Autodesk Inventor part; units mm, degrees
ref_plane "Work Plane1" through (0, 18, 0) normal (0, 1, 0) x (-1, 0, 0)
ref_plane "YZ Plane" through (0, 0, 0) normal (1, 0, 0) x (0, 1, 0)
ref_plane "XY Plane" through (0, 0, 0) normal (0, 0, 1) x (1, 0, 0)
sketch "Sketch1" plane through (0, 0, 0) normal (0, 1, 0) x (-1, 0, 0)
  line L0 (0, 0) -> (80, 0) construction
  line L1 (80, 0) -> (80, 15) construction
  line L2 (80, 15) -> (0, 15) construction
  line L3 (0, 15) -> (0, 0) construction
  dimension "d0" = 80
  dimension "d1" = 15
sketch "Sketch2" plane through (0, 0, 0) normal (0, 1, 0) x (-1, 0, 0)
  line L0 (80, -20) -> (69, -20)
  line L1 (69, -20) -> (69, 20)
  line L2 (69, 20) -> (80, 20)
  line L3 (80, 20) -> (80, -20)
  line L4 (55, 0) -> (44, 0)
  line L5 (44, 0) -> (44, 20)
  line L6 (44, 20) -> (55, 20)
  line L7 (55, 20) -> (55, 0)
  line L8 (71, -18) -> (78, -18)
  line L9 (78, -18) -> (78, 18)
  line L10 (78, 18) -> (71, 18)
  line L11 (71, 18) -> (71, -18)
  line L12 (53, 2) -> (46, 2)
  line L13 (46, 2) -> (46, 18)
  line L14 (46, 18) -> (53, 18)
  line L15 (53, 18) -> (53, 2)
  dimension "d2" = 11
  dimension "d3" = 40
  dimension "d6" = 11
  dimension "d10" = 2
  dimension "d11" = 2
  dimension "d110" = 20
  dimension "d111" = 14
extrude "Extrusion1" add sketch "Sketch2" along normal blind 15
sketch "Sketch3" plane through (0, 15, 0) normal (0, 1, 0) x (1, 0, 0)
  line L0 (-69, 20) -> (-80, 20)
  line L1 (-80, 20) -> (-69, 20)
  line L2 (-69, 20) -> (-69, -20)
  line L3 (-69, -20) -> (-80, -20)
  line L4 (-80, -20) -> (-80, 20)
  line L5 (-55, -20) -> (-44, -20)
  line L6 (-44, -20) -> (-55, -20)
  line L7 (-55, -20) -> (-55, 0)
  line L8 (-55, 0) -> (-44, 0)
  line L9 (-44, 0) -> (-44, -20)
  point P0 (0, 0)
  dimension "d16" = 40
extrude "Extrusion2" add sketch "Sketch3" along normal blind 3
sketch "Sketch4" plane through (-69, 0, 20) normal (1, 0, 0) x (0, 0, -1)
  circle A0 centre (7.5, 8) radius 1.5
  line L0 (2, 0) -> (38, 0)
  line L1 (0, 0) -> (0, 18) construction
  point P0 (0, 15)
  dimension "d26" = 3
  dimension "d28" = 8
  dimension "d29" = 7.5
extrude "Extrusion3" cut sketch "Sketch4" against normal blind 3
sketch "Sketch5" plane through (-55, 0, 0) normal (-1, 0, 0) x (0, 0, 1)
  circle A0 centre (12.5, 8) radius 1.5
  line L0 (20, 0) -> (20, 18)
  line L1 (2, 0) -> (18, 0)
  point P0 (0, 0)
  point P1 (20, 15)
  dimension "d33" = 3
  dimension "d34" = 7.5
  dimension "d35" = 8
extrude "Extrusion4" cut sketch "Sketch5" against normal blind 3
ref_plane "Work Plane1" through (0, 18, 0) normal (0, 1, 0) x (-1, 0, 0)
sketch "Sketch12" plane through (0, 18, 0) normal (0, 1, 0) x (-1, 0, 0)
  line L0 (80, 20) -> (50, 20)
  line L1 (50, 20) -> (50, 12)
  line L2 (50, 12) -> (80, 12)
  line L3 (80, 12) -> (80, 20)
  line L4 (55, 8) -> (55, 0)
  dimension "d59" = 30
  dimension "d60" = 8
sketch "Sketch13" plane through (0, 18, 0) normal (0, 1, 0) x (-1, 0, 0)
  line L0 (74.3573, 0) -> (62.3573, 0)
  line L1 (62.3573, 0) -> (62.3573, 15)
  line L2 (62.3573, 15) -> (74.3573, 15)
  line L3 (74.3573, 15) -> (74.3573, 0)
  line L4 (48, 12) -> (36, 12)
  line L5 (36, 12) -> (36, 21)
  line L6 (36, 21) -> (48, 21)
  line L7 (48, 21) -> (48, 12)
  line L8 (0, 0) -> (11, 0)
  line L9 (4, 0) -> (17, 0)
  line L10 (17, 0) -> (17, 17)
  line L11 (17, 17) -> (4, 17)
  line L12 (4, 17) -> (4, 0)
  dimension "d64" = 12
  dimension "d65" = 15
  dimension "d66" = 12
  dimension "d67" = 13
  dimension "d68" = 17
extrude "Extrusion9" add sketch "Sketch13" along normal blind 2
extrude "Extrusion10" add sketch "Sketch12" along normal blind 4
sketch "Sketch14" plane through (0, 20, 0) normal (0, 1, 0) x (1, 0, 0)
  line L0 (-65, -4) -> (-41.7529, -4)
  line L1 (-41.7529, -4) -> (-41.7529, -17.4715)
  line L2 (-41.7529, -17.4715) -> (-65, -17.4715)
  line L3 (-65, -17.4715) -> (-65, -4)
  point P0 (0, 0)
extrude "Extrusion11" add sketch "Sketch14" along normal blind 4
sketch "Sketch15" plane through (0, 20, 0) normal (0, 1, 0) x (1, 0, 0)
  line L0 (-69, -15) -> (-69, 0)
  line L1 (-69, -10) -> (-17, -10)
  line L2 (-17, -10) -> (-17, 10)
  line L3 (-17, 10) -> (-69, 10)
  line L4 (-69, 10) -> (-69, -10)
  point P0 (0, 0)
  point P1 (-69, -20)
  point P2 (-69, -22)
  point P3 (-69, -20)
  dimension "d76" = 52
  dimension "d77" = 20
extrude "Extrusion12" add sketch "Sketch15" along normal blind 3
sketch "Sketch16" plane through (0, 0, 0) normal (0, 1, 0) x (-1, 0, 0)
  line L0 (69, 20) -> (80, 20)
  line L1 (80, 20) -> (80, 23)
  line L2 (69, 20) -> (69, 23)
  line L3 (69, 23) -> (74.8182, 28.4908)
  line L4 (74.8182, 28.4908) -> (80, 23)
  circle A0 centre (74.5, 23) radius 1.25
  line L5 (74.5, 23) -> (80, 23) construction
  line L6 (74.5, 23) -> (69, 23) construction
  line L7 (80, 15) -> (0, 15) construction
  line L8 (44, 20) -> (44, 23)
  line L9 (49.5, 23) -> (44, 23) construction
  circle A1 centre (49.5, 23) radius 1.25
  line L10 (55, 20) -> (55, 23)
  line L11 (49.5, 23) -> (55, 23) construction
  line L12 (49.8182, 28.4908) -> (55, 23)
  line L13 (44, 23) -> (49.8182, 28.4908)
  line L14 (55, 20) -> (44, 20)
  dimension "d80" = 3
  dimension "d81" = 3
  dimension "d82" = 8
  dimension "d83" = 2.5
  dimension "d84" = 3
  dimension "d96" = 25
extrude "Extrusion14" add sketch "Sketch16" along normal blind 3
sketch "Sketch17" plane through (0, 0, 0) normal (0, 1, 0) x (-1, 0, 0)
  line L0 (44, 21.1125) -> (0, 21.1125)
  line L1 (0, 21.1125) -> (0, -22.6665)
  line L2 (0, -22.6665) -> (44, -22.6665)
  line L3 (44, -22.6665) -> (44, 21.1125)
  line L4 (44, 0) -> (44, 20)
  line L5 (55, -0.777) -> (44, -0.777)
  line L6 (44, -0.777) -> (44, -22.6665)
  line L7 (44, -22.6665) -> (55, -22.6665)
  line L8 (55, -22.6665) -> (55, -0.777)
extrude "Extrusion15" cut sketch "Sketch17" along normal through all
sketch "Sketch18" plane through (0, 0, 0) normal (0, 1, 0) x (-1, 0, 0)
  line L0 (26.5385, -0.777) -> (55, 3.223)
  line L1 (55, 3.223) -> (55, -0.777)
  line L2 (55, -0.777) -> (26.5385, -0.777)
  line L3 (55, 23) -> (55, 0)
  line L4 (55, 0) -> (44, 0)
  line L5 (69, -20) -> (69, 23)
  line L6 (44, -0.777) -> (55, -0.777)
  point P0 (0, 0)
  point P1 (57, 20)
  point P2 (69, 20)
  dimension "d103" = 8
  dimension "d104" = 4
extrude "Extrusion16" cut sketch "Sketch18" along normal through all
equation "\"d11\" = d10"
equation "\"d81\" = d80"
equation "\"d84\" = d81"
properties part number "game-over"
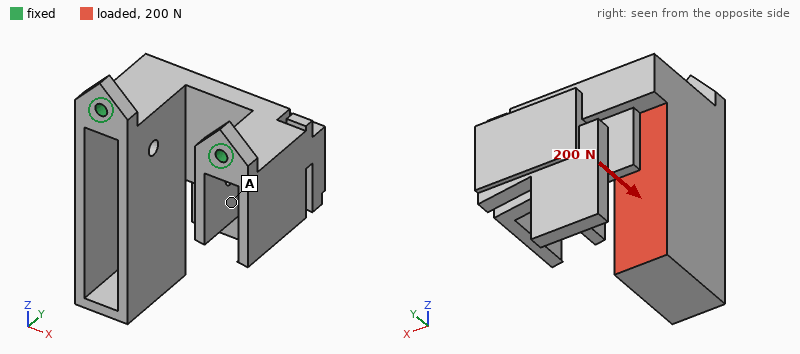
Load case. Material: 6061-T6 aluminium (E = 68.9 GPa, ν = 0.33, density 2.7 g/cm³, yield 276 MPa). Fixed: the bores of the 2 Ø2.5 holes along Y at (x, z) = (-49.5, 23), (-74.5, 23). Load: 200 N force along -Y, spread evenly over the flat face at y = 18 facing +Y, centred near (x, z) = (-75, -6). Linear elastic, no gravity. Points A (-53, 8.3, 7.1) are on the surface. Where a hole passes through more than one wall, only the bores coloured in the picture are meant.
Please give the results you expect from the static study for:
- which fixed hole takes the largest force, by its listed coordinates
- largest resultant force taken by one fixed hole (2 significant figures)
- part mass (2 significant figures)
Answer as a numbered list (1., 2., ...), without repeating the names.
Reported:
1. (-74.5, 23)
2. 200 N
3. 25 g
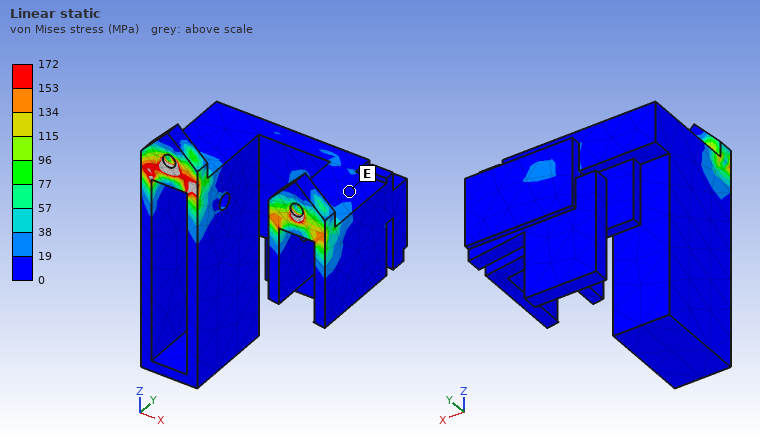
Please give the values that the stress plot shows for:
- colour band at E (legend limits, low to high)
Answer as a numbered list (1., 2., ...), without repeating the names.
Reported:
1. 0 to 19 MPa
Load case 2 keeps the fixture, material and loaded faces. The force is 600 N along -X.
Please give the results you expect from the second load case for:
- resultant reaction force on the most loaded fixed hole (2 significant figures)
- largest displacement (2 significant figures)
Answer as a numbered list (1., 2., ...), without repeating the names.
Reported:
1. 580 N
2. 0.49 mm
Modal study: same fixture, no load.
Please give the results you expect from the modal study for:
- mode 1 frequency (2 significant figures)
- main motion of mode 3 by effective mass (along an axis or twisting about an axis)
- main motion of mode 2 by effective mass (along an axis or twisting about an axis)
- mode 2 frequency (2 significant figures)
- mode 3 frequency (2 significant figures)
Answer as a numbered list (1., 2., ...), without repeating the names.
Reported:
1. 1000 Hz
2. along X
3. along X
4. 1900 Hz
5. 4900 Hz
